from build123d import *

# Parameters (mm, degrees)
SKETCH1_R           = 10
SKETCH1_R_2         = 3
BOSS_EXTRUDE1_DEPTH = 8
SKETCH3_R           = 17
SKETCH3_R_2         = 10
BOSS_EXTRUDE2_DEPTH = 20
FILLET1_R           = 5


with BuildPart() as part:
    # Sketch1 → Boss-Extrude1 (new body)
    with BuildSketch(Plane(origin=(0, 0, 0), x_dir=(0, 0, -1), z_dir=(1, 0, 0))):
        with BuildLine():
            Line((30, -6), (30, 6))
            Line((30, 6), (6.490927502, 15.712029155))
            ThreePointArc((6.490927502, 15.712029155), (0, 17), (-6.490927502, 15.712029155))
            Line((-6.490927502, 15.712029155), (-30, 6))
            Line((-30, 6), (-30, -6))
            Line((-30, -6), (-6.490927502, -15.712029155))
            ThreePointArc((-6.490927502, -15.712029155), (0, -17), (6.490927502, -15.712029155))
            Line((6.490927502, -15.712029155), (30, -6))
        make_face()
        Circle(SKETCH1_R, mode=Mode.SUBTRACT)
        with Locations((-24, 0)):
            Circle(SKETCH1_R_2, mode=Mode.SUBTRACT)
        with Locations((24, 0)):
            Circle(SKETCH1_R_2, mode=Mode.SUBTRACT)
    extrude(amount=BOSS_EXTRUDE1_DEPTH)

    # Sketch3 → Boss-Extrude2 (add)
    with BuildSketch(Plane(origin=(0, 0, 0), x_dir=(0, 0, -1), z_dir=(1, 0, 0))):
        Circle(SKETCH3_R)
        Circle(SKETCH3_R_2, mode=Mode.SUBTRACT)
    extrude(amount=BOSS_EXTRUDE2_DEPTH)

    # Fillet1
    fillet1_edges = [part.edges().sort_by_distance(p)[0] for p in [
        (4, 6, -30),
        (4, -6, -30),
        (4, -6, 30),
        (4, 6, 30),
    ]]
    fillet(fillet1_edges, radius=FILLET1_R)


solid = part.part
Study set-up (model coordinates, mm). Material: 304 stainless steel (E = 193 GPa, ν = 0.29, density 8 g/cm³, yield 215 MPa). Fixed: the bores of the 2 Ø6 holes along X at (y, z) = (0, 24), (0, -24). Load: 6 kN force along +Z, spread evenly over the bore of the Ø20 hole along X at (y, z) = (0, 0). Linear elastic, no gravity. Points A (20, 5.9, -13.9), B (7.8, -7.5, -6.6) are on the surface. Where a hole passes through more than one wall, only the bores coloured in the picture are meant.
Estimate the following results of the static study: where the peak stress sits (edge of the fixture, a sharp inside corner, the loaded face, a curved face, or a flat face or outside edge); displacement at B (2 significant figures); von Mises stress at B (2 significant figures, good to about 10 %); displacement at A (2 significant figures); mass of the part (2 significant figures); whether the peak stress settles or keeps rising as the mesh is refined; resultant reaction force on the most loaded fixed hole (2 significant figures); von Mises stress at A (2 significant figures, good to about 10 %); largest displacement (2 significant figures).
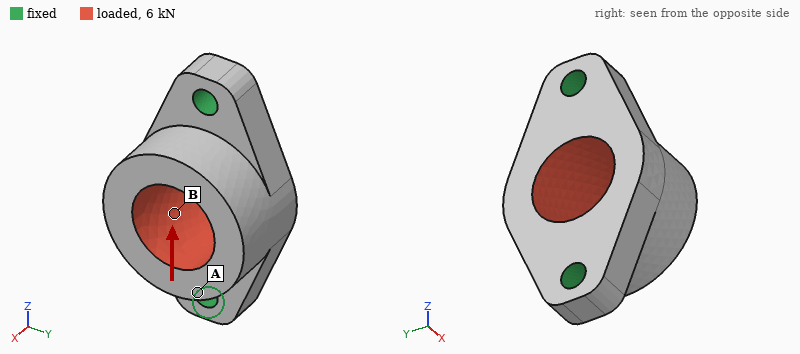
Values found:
edge of the fixture
2.1 µm
19 MPa
3.6 µm
130 g
keeps rising
3.1 kN
8.5 MPa
3.7 µm
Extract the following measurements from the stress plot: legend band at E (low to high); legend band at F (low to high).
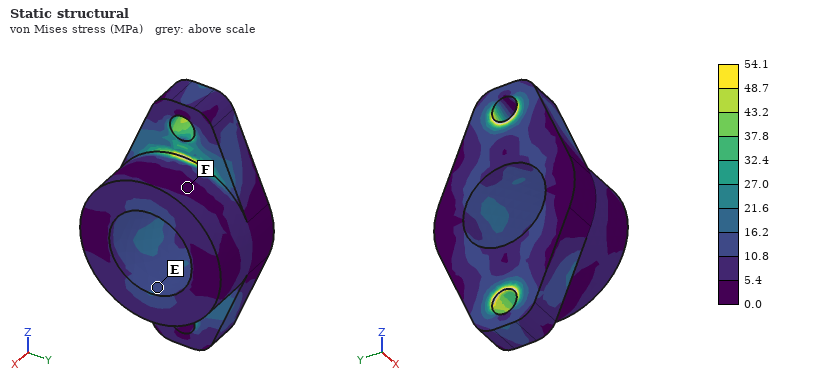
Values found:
10.8 to 16.2 MPa
0.0 to 5.4 MPa
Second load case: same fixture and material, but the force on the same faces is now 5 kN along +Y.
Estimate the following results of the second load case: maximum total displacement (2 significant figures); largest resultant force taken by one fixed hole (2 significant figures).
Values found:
19 µm
2.5 kN
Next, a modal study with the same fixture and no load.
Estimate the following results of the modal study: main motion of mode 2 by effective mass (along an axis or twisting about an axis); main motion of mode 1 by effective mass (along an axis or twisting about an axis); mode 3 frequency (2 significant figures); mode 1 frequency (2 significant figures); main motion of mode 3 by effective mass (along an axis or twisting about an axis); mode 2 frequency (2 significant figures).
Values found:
along X
along Y
22 kHz
8100 Hz
along Y
14 kHz
